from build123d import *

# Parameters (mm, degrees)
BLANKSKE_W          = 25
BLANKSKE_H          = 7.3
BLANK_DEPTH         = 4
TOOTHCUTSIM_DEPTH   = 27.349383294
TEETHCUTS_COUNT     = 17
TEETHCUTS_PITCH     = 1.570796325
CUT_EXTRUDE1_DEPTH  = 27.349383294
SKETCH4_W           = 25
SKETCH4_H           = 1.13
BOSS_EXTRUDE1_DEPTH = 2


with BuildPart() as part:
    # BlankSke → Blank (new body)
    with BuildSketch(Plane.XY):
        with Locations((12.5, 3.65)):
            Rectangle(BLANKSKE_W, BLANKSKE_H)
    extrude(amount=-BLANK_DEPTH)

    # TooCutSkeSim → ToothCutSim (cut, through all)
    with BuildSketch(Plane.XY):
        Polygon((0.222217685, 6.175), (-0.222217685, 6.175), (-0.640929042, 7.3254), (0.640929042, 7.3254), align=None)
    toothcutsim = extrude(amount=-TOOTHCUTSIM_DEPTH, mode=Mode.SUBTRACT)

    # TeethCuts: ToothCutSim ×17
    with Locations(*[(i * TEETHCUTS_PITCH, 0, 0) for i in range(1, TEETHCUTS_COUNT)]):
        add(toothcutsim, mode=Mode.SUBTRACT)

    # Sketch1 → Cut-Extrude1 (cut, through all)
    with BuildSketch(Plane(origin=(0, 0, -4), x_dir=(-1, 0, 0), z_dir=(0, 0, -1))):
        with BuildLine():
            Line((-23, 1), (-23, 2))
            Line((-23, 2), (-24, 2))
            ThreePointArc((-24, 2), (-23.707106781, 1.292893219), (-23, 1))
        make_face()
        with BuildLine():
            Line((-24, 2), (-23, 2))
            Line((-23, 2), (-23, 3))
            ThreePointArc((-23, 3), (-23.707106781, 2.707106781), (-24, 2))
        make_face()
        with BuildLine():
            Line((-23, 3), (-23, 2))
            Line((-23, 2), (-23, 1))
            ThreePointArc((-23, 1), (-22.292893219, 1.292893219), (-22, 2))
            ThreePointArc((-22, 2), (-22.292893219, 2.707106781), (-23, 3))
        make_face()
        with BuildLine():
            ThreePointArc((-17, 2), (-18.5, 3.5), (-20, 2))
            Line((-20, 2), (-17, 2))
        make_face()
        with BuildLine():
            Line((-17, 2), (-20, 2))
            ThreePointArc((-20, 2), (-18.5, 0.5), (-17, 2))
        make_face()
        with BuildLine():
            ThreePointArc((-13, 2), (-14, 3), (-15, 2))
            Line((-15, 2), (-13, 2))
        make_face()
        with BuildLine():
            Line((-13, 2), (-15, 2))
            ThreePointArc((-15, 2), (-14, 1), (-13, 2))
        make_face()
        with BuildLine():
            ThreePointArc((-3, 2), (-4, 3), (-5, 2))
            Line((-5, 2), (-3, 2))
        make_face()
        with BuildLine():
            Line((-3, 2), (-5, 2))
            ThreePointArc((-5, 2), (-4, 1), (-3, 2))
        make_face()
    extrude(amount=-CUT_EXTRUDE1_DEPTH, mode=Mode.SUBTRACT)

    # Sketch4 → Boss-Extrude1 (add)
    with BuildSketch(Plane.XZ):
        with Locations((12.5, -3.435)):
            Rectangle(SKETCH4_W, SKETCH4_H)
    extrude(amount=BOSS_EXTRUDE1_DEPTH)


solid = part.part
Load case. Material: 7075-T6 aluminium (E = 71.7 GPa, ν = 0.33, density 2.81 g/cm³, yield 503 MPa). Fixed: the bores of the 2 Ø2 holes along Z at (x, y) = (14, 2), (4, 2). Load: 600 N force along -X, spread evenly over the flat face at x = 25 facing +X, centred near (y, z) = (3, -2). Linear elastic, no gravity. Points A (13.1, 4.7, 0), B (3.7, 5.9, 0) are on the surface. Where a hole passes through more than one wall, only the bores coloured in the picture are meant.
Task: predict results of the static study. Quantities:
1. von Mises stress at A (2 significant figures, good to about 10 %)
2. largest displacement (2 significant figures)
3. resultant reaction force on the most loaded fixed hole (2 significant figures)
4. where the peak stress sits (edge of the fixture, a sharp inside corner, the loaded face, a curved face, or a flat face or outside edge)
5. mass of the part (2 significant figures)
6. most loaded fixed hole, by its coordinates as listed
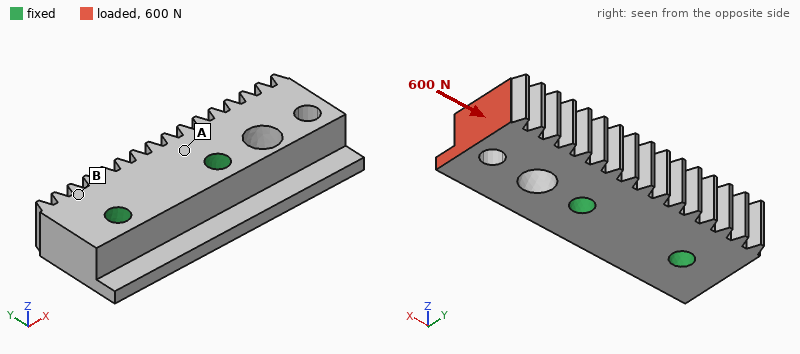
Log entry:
16 MPa
7.6 µm
510 N
a curved face
1.9 g
(14, 2)
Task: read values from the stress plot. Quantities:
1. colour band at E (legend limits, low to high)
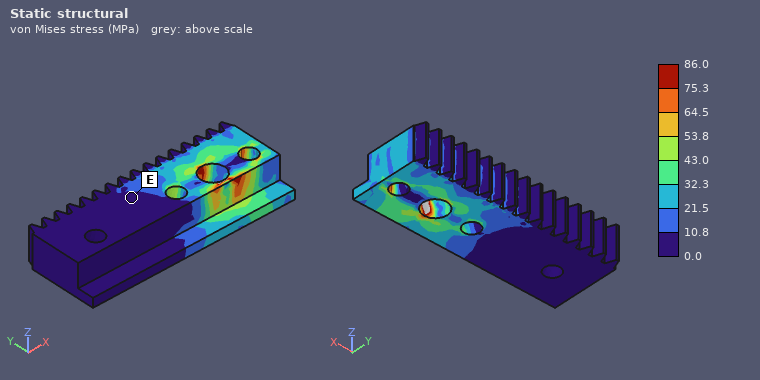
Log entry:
0.0 to 10.8 MPa
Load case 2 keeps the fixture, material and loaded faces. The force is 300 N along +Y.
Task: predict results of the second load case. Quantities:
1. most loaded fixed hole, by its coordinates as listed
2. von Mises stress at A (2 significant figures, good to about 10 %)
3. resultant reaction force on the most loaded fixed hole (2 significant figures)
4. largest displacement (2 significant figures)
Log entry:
(14, 2)
37 MPa
510 N
44 µm
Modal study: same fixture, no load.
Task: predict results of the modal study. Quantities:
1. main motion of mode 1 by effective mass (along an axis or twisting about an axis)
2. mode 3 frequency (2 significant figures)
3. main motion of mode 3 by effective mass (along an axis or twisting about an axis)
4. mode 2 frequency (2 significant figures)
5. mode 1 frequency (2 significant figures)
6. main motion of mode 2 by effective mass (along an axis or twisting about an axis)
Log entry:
along Z
41 kHz
twisting about X
28 kHz
21 kHz
along Y
